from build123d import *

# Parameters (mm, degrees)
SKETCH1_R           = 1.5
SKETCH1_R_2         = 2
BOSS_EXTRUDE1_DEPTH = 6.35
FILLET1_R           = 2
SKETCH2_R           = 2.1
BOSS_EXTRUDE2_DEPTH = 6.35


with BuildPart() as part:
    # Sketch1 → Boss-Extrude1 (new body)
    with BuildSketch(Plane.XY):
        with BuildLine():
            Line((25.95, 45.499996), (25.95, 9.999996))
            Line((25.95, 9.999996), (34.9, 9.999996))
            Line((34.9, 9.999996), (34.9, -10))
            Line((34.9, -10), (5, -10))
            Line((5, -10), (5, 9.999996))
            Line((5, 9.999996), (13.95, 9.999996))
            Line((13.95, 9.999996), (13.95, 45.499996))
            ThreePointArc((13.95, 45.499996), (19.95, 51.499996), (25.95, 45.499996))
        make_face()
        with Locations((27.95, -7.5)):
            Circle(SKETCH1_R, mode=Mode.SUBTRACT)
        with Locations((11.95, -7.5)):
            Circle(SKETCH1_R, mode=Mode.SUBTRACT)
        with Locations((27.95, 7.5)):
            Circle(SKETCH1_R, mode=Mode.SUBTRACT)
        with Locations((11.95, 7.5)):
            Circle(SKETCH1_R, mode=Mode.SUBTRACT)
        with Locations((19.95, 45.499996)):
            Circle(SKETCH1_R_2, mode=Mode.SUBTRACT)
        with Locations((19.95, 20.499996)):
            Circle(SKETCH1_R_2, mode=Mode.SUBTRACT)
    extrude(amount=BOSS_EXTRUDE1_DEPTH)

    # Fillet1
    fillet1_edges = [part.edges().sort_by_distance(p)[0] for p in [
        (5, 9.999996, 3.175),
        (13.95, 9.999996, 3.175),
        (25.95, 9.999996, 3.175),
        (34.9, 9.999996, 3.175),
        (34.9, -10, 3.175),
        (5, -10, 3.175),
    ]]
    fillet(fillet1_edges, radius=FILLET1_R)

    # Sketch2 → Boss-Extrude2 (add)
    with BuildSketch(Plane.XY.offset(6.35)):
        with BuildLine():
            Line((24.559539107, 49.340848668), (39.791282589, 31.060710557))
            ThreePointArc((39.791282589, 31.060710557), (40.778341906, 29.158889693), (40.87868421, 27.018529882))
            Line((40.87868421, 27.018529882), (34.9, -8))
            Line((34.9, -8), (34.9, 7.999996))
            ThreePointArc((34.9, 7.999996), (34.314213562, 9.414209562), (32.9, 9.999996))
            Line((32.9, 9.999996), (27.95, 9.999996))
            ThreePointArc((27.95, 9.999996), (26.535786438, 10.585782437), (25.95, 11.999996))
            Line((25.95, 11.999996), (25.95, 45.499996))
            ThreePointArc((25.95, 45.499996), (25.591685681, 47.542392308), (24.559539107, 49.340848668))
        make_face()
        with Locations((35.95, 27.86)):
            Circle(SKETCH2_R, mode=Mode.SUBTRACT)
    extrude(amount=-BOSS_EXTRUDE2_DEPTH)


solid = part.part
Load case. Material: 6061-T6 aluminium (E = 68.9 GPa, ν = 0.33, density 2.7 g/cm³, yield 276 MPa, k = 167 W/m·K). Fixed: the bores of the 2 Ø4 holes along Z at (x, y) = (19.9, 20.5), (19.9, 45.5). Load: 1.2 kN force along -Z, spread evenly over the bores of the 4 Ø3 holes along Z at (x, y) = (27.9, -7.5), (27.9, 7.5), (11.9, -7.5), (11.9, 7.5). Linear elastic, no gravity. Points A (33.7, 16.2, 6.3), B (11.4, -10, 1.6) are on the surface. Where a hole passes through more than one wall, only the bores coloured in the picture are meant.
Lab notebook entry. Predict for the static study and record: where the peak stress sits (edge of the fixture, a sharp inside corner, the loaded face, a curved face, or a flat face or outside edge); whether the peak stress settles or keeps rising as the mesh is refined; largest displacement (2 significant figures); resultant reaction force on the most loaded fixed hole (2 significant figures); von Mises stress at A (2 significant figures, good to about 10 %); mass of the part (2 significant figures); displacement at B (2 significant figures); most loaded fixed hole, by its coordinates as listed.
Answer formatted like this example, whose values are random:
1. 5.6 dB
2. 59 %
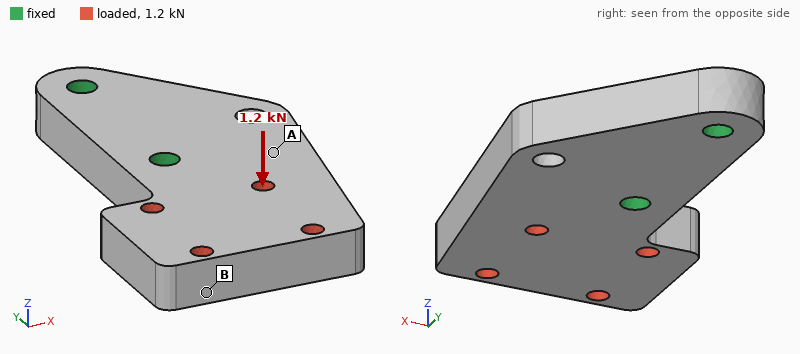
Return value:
1. edge of the fixture
2. keeps rising
3. 0.23 mm
4. 1.5 kN
5. 65 MPa
6. 25 g
7. 0.23 mm
8. (19.9, 20.5)
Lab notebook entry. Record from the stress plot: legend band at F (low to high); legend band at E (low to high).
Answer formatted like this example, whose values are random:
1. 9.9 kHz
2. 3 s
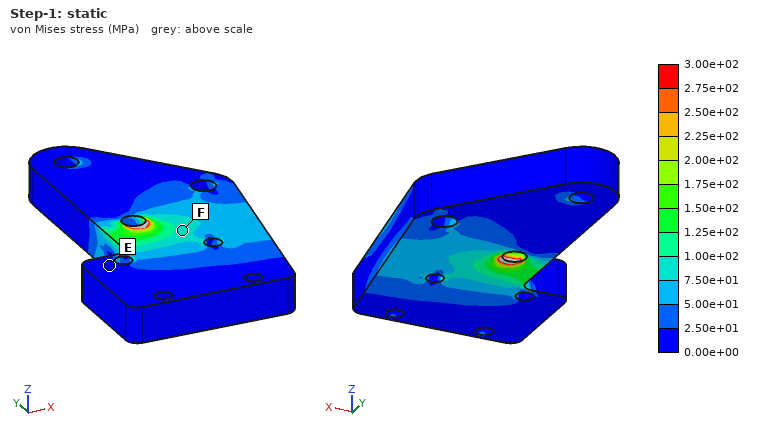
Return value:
1. 7.50e+01 to 1.00e+02 MPa
2. 0.00e+00 to 2.50e+01 MPa
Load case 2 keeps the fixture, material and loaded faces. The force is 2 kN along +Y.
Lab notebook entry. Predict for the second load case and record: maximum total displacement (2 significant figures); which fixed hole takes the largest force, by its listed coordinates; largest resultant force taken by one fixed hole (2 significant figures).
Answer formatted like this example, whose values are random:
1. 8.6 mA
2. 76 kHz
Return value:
1. 16 µm
2. (19.9, 20.5)
3. 1.8 kN
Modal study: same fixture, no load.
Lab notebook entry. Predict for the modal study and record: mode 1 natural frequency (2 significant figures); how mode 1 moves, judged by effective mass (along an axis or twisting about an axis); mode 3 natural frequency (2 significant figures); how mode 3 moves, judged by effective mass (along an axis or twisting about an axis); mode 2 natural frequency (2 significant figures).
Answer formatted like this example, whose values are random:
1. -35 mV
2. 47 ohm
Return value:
1. 4500 Hz
2. along Z
3. 9400 Hz
4. along X
5. 7600 Hz
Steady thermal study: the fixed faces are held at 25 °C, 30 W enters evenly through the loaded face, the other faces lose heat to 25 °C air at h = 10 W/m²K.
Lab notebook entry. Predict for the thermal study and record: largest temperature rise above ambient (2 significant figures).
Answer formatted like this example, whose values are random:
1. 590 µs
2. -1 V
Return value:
1. 30 K
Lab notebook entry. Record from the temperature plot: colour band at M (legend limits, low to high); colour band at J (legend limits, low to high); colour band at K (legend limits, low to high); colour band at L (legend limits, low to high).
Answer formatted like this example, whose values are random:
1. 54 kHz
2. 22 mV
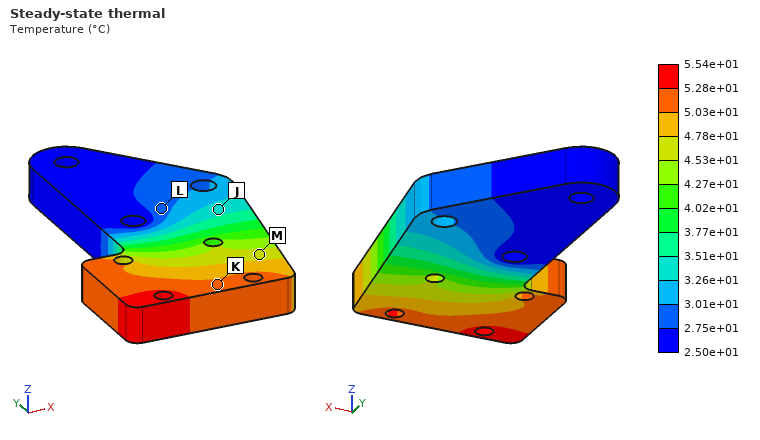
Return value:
1. 4.53e+01 to 4.78e+01 °C
2. 3.26e+01 to 3.51e+01 °C
3. 5.03e+01 to 5.28e+01 °C
4. 2.75e+01 to 3.01e+01 °C
